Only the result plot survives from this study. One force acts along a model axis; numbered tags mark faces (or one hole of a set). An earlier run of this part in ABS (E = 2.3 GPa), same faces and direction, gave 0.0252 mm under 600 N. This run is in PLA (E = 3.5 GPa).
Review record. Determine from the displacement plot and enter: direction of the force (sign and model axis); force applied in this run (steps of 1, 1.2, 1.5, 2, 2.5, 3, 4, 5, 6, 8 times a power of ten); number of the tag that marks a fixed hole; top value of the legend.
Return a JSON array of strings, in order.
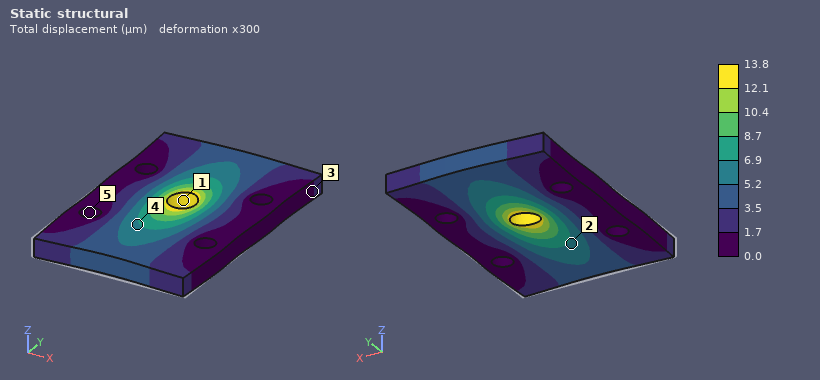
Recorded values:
["+Y", "500 N", "5", "13.8 µm"]
